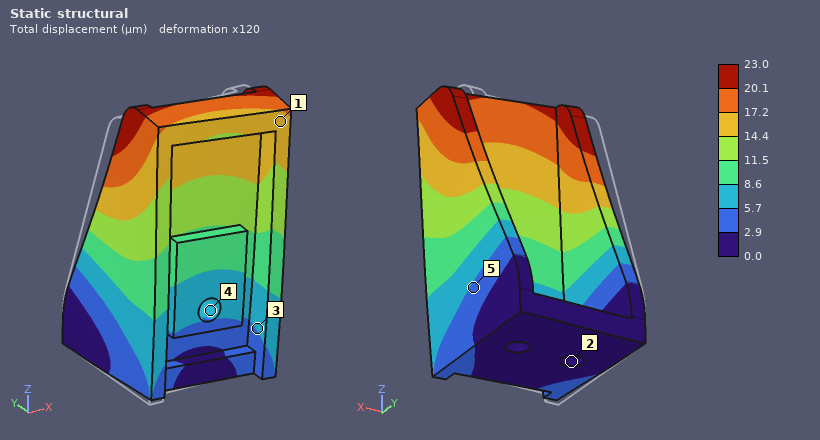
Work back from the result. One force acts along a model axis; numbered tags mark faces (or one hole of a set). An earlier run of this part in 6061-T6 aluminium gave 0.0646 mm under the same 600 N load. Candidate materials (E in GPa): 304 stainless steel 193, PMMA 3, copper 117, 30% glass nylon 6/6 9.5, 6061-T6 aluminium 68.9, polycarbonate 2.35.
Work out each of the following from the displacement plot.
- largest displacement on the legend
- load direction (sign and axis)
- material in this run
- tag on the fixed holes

23.0 µm
+X
304 stainless steel
2
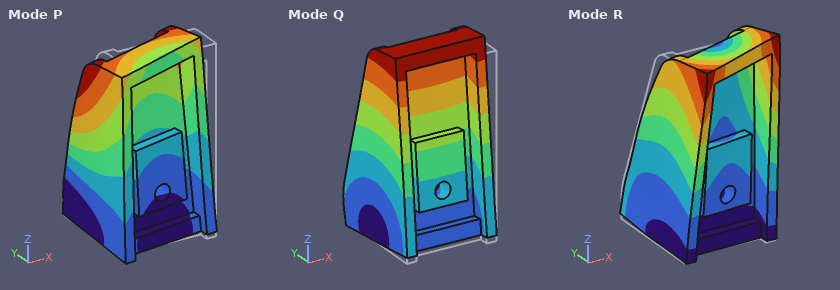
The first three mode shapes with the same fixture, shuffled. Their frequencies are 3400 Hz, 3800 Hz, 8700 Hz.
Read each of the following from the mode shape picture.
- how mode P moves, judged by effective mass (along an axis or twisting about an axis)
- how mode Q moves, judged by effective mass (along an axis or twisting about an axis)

along X
along Y
